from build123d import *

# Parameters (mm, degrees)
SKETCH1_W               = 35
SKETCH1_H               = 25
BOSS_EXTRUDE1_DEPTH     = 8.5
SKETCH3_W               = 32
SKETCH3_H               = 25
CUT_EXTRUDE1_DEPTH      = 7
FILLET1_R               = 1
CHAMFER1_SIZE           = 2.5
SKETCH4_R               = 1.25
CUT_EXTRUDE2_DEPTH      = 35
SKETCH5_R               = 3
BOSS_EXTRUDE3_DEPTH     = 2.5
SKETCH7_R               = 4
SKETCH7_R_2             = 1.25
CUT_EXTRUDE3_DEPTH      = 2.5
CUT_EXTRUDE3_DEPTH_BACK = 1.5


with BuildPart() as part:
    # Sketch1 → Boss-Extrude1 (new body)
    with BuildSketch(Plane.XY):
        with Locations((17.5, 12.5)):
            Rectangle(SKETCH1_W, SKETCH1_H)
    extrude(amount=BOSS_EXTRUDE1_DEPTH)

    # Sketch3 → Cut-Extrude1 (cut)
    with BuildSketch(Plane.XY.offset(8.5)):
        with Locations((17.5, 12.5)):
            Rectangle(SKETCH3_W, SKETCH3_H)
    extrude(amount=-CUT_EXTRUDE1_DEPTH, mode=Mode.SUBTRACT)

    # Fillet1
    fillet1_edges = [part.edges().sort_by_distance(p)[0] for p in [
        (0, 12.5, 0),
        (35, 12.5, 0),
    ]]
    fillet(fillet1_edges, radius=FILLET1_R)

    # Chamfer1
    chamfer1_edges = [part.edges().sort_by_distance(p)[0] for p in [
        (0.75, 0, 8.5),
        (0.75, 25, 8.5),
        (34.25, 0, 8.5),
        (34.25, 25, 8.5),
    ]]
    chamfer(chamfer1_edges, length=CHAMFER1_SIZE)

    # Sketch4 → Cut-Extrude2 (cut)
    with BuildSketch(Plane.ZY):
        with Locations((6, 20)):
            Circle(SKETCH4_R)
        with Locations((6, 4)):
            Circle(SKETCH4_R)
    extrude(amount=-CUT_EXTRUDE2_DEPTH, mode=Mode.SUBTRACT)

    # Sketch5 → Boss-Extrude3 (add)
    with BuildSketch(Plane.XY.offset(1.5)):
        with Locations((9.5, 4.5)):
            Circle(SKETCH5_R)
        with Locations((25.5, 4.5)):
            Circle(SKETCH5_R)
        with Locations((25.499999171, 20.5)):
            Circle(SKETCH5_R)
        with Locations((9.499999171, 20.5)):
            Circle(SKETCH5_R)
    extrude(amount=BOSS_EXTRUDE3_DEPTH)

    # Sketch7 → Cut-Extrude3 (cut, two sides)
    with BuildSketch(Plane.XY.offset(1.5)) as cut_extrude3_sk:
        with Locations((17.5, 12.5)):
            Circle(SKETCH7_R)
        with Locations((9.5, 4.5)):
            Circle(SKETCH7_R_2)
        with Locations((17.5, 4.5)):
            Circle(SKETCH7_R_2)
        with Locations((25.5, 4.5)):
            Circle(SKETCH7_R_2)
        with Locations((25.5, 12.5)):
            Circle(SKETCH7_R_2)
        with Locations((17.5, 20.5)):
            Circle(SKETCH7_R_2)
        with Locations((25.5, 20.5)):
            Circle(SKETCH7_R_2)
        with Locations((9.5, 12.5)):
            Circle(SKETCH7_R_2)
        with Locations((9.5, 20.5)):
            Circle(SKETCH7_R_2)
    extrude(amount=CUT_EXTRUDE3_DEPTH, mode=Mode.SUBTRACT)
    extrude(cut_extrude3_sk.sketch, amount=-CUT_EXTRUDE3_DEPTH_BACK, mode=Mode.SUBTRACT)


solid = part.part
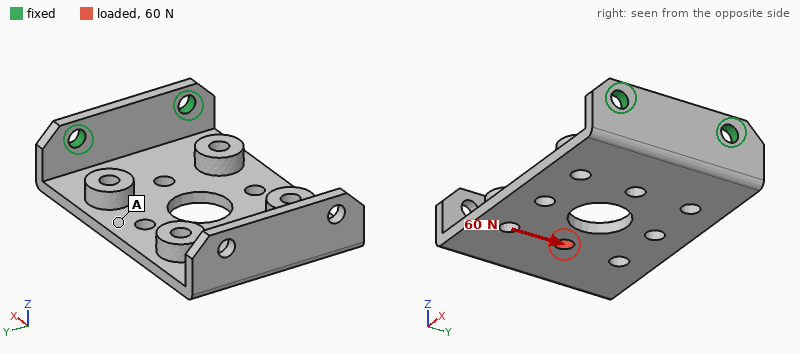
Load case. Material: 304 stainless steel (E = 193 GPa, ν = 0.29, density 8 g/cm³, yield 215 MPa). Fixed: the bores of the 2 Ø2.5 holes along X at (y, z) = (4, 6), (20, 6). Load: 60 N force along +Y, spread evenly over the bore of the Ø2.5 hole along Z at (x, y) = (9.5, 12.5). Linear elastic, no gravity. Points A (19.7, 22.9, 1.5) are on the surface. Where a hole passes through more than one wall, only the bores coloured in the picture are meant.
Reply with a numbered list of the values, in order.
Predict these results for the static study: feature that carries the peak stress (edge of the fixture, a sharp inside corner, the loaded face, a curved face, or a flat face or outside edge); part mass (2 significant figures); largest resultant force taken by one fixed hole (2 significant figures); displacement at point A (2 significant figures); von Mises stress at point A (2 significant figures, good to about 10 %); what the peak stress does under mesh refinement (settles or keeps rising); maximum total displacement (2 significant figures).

1. edge of the fixture
2. 15 g
3. 93 N
4. 12 µm
5. 8.5 MPa
6. keeps rising
7. 26 µm
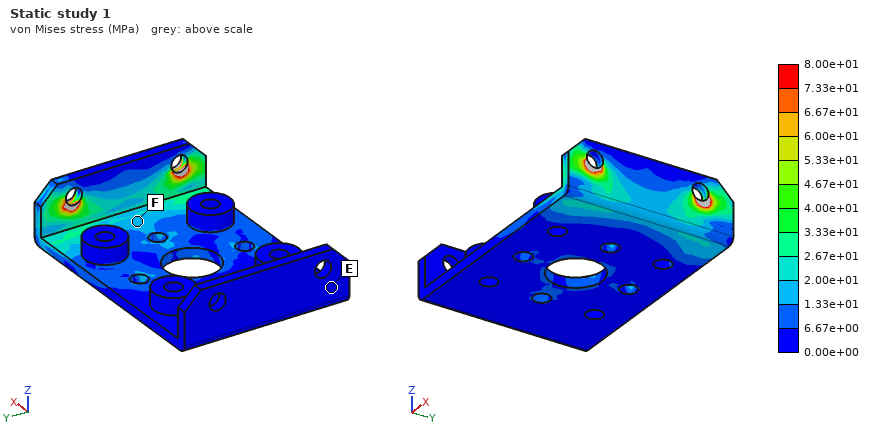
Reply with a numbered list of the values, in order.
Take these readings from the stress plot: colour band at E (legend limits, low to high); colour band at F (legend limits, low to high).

1. 0.00e+00 to 6.67e+00 MPa
2. 1.33e+01 to 2.00e+01 MPa
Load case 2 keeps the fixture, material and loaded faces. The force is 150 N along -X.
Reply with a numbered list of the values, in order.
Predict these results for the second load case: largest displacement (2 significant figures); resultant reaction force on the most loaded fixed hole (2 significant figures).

1. 52 µm
2. 79 N
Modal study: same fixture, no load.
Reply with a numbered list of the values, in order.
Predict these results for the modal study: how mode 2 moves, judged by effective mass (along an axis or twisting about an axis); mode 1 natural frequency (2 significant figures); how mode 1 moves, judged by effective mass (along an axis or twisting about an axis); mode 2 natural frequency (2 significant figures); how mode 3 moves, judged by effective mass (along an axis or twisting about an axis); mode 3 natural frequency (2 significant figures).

1. along Y
2. 630 Hz
3. along Z
4. 2200 Hz
5. along Y
6. 3600 Hz
